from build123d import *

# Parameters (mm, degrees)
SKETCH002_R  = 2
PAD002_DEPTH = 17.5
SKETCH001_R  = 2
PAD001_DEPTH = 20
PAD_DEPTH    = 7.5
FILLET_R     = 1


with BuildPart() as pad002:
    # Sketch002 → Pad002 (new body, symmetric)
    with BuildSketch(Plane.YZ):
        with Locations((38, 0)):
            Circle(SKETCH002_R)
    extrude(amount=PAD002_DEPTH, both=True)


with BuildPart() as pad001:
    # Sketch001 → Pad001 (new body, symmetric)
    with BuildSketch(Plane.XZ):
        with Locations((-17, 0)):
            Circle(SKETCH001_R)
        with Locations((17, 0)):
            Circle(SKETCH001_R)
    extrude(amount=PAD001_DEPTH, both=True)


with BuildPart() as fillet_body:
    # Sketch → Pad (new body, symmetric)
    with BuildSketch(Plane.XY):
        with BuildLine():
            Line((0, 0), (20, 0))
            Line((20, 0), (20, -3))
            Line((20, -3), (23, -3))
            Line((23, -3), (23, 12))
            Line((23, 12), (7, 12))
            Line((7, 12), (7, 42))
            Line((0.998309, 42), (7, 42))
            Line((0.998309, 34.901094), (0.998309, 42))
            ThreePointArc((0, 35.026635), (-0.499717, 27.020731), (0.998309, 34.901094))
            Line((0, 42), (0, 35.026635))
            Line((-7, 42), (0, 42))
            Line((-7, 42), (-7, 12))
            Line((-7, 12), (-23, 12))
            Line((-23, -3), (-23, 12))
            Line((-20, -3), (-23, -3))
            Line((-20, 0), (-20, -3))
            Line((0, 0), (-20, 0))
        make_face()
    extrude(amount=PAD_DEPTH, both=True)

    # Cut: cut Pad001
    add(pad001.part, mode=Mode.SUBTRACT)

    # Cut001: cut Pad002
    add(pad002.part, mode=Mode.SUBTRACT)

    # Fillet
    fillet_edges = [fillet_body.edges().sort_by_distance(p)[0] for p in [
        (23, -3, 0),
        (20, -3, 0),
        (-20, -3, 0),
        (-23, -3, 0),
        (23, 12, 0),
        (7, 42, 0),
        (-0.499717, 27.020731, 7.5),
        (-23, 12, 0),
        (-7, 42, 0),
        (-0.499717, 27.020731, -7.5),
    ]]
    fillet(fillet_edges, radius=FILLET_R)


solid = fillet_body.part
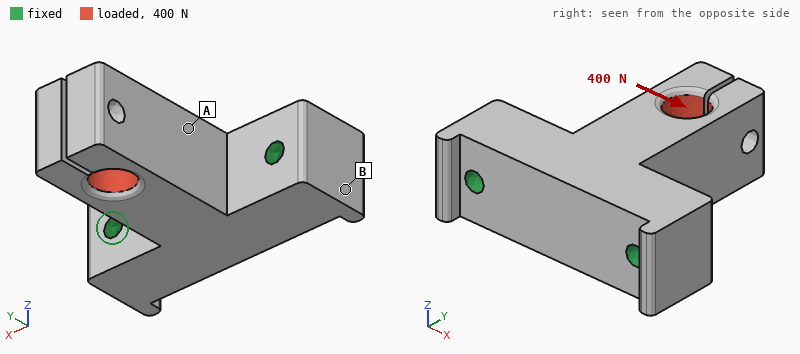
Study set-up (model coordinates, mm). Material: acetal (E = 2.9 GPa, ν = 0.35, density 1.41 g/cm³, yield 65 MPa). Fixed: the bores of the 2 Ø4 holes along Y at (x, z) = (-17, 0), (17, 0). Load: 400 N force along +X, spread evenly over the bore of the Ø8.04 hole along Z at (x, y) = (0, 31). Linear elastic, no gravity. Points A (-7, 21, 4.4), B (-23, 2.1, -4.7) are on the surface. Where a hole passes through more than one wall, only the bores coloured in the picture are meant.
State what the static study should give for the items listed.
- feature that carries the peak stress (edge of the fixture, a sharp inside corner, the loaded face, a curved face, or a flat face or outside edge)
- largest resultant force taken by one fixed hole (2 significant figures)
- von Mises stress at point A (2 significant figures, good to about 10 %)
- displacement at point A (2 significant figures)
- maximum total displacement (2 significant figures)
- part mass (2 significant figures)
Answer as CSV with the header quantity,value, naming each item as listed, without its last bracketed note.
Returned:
quantity,value
feature that carries the peak stress,the loaded face
largest resultant force taken by one fixed hole,400 N
von Mises stress at point A,8.9 MPa
displacement at point A,0.13 mm
maximum total displacement,0.65 mm
part mass,19 g
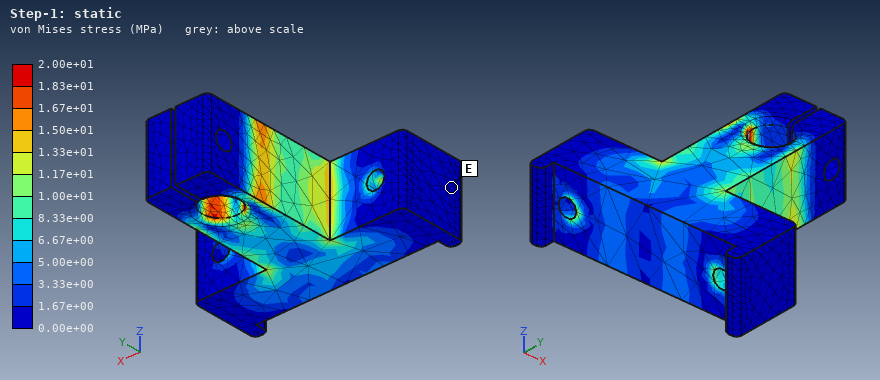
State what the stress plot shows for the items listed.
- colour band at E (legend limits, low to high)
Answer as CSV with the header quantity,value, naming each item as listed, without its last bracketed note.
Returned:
quantity,value
colour band at E,0.00e+00 to 1.67e+00 MPa
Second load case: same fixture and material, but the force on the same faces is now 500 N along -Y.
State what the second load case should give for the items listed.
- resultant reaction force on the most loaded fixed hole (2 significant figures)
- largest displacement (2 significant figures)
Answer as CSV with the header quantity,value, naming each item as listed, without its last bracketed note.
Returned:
quantity,value
resultant reaction force on the most loaded fixed hole,260 N
largest displacement,0.30 mm
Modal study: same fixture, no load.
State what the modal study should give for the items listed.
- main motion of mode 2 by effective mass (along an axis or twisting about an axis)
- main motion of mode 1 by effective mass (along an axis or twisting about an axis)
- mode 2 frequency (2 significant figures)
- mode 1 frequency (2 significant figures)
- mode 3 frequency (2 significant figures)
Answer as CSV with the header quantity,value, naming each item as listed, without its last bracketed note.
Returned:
quantity,value
main motion of mode 2 by effective mass,along X
main motion of mode 1 by effective mass,along Z
mode 2 frequency,1900 Hz
mode 1 frequency,1800 Hz
mode 3 frequency,2400 Hz
